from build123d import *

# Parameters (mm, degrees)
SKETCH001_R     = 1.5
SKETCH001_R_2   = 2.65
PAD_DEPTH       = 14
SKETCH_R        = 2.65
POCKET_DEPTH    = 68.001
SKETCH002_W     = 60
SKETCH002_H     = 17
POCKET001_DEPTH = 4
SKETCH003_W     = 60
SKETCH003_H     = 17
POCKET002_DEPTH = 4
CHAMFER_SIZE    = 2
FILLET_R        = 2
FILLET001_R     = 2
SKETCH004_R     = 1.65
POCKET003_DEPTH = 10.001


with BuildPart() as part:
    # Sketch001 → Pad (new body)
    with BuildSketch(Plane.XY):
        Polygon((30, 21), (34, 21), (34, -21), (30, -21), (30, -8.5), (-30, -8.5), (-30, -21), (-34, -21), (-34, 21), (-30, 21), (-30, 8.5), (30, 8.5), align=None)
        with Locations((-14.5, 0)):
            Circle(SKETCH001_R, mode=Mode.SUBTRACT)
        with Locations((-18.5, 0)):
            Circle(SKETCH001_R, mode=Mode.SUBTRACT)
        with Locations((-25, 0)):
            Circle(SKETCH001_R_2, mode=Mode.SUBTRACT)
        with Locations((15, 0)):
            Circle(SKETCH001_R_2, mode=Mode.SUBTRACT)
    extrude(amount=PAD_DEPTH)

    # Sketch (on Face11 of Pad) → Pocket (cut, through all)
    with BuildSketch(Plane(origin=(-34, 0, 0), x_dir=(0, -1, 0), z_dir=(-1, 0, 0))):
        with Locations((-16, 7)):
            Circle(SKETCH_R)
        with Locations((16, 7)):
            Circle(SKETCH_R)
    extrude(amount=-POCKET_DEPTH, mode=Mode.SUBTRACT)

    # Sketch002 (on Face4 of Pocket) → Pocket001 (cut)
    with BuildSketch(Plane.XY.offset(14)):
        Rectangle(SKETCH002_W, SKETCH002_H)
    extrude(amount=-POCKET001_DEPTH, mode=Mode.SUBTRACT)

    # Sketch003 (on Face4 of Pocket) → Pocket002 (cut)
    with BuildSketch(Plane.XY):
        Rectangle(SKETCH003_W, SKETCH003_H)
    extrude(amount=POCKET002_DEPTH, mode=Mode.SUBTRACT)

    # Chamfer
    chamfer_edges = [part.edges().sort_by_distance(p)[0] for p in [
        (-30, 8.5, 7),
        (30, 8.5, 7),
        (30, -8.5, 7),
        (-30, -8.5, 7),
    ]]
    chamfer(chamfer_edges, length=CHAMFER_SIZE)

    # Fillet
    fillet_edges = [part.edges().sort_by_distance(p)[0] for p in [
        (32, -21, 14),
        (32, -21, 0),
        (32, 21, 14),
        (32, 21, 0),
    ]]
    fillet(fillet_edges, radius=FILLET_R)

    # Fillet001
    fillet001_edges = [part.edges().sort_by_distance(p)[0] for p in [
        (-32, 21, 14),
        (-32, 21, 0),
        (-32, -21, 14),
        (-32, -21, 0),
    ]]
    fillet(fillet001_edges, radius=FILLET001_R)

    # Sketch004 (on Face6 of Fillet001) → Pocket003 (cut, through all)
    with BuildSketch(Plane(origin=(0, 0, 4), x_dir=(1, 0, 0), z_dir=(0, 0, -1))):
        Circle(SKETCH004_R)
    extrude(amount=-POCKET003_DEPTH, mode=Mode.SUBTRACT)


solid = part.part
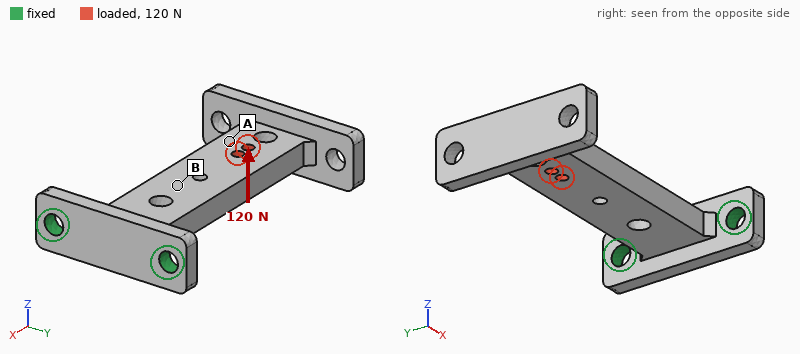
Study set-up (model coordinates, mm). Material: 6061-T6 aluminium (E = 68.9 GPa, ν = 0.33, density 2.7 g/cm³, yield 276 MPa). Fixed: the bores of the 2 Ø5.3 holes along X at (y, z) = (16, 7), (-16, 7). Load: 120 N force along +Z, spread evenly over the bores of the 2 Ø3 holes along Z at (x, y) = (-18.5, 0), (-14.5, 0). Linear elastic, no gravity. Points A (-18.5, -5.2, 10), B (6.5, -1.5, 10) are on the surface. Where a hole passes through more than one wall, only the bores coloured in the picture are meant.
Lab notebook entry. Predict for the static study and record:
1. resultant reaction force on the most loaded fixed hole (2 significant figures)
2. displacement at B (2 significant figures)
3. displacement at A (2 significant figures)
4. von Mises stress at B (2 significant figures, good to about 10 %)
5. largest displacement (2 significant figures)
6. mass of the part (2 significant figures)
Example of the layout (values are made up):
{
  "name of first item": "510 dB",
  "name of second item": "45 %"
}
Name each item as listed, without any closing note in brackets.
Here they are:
{
  "resultant reaction force on the most loaded fixed hole": "60 N",
  "displacement at B": "0.14 mm",
  "displacement at A": "0.37 mm",
  "von Mises stress at B": "24 MPa",
  "largest displacement": "0.52 mm",
  "mass of the part": "27 g"
}
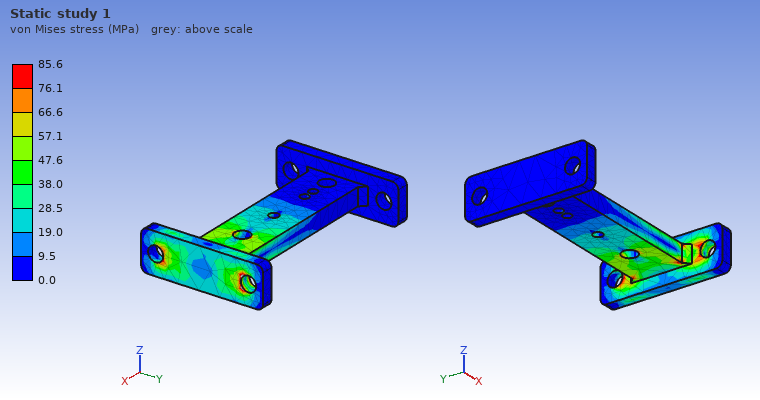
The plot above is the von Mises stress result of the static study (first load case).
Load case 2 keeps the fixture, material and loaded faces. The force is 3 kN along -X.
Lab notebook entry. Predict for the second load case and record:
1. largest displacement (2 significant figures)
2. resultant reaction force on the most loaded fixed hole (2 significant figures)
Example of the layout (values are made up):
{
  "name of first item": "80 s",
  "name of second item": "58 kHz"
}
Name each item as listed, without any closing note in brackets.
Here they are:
{
  "largest displacement": "49 µm",
  "resultant reaction force on the most loaded fixed hole": "1.6 kN"
}
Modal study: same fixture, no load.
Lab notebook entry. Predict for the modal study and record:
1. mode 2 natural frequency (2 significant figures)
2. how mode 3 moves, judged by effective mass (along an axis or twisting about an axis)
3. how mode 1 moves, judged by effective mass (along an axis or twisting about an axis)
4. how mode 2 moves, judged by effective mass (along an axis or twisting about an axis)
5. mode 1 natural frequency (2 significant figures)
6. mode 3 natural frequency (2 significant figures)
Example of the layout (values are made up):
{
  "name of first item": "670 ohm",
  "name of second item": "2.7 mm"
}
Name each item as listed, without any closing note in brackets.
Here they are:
{
  "mode 2 natural frequency": "1900 Hz",
  "how mode 3 moves, judged by effective mass": "twisting about X",
  "how mode 1 moves, judged by effective mass": "along Z",
  "how mode 2 moves, judged by effective mass": "along Y",
  "mode 1 natural frequency": "650 Hz",
  "mode 3 natural frequency": "2900 Hz"
}
